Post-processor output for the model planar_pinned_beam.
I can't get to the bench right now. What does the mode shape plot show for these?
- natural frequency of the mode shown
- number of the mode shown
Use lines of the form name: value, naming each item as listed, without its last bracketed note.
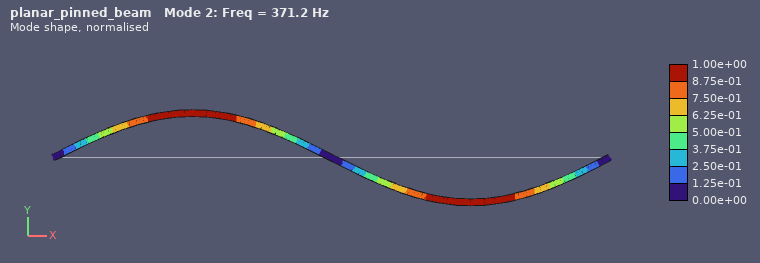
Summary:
natural frequency of the mode shown: 371.2 Hz
number of the mode shown: 2
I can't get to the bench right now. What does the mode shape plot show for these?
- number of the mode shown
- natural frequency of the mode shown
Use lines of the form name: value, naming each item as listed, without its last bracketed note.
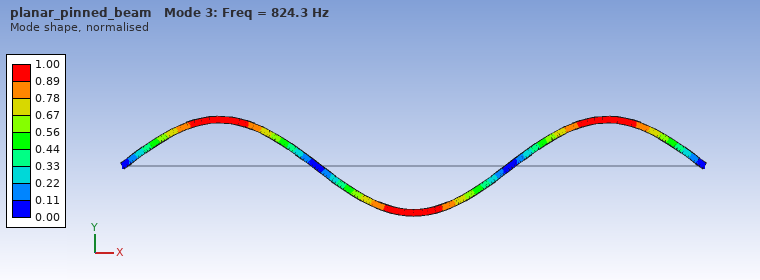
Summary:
number of the mode shown: 3
natural frequency of the mode shown: 824.3 Hz
